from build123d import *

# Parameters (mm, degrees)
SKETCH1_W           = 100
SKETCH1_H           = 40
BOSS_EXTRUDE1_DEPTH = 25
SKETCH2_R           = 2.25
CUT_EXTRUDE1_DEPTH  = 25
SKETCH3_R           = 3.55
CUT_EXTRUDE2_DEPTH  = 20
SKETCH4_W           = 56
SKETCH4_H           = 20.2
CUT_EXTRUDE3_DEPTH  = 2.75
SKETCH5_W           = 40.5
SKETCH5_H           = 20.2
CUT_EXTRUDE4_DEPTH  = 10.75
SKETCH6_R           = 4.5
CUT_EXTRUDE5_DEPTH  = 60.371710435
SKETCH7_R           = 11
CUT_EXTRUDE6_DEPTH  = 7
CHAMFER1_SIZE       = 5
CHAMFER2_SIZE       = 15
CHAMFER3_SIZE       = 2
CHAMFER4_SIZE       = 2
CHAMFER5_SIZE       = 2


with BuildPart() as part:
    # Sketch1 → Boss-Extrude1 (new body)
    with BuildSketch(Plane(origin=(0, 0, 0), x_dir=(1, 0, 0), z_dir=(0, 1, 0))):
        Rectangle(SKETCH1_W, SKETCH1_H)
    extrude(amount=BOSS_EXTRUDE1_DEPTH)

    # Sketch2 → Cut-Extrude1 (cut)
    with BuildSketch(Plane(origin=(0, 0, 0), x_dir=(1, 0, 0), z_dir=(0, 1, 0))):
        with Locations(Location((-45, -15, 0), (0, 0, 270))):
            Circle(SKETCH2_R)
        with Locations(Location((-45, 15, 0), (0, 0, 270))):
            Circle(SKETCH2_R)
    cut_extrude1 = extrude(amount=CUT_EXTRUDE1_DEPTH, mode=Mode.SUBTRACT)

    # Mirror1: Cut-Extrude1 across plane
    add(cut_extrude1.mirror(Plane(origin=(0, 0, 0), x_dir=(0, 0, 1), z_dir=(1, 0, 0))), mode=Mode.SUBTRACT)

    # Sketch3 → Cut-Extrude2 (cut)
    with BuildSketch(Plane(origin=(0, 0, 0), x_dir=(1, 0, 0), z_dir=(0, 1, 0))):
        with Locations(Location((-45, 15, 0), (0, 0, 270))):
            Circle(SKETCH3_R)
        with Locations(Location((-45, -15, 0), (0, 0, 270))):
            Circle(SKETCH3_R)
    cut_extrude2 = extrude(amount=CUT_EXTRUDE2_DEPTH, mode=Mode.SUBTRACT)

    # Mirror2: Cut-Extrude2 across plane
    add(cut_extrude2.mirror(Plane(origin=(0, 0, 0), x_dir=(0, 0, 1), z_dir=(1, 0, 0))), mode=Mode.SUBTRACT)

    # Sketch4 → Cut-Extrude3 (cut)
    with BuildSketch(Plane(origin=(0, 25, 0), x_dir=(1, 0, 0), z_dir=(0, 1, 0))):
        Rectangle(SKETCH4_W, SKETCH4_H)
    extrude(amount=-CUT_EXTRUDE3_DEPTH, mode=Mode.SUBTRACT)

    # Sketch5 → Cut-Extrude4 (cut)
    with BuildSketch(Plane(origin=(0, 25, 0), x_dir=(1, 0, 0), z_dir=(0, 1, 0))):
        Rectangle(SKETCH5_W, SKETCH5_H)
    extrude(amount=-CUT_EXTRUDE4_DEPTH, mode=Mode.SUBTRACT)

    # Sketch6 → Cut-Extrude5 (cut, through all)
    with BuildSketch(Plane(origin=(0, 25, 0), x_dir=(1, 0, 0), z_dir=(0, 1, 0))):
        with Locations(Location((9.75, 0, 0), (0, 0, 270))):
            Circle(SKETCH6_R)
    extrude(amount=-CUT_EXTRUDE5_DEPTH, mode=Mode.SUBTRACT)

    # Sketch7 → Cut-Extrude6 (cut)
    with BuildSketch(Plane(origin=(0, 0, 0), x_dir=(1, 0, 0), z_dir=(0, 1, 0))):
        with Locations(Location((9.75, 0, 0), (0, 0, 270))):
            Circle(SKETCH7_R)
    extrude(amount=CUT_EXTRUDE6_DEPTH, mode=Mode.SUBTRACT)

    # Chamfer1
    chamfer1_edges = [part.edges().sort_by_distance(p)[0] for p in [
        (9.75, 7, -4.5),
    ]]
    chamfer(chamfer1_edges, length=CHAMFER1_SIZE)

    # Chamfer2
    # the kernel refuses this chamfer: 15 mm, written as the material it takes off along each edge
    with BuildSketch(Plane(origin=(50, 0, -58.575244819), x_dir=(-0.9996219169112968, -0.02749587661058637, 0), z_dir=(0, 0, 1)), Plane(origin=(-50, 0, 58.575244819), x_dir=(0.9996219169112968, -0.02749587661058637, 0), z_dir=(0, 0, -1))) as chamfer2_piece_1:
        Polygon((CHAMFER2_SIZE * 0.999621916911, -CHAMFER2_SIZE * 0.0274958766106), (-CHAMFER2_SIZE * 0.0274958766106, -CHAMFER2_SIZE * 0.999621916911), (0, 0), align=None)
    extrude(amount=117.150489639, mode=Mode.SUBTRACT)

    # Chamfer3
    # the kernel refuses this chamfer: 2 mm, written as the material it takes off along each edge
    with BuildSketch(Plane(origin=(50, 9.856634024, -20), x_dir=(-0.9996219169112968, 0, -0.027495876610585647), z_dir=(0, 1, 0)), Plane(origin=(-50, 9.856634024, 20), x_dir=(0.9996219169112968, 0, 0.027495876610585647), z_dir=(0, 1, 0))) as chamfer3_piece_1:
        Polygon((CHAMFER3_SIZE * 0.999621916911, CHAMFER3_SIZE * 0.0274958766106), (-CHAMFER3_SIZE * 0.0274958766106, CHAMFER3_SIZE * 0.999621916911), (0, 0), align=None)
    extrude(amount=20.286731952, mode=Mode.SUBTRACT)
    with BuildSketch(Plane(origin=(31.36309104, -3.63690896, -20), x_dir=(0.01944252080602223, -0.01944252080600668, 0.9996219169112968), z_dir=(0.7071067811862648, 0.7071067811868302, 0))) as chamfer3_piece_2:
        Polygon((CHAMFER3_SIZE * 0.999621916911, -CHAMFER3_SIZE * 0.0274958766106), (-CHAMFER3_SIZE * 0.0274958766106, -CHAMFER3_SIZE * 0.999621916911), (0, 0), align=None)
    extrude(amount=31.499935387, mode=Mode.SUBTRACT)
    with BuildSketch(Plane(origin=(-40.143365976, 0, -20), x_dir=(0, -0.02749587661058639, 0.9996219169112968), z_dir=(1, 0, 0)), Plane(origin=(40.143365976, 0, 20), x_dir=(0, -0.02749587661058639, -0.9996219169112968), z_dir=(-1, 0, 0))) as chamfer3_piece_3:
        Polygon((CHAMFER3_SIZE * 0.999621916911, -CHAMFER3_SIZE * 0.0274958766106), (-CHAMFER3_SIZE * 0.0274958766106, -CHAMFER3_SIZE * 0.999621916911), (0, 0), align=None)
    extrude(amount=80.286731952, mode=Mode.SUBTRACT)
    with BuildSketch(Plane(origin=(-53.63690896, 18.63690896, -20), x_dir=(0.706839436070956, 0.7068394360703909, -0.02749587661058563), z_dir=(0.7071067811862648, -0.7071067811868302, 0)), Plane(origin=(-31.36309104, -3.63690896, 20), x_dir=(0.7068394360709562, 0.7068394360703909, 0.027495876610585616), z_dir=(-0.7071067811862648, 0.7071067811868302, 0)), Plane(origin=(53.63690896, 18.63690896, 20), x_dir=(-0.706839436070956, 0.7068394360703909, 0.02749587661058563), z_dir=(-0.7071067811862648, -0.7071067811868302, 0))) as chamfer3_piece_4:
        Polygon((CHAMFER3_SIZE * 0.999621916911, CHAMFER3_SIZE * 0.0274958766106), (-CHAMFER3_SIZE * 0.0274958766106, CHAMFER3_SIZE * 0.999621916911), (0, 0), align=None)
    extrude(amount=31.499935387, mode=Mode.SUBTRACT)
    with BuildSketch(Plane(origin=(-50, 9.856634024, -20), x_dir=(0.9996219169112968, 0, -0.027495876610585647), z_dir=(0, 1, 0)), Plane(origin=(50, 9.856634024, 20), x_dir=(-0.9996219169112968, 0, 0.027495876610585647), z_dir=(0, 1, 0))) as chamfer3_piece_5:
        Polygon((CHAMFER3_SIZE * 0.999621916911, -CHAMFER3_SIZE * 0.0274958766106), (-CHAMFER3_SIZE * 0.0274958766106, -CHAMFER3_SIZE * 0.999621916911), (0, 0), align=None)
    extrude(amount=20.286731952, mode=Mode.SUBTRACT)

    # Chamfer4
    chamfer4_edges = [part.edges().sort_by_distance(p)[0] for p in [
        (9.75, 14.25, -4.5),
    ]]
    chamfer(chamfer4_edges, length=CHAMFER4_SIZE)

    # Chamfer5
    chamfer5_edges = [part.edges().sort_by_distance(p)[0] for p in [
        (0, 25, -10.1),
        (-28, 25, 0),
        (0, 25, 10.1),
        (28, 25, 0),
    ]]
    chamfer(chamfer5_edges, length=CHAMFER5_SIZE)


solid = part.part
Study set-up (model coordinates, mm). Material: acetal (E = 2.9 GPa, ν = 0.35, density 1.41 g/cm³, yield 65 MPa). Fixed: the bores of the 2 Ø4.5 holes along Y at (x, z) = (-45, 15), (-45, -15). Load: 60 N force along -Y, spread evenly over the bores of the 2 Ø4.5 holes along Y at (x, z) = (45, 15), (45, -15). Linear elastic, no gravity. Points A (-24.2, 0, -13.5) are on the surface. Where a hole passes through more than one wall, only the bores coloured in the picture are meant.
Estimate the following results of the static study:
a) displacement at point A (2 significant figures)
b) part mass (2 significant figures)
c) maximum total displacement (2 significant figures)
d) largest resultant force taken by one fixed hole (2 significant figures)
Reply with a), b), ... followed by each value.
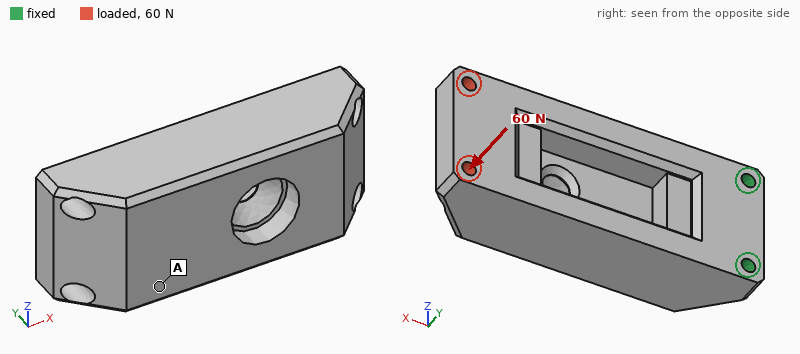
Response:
a) 0.37 mm
b) 110 g
c) 1.3 mm
d) 33 N
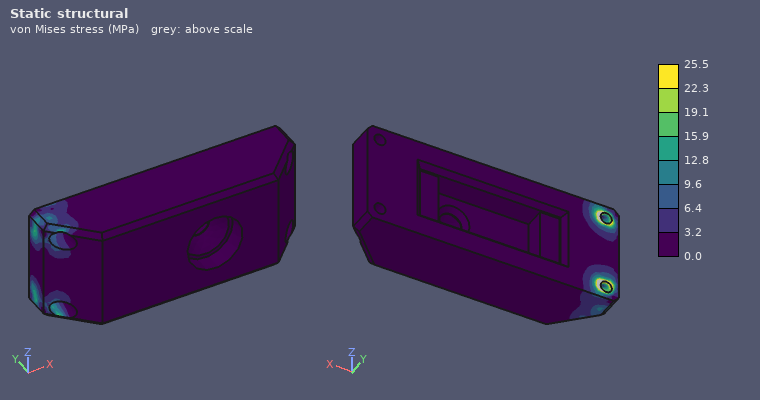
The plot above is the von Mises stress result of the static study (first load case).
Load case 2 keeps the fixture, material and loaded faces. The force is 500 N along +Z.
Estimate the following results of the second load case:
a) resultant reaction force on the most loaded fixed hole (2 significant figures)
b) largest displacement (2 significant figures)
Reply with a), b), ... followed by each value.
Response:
a) 1.4 kN
b) 1.2 mm
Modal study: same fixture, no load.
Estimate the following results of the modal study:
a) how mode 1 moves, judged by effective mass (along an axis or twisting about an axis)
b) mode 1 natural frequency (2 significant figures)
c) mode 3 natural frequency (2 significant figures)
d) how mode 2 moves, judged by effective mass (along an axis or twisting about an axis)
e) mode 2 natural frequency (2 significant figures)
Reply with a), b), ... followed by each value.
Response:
a) along Y
b) 190 Hz
c) 1400 Hz
d) along Z
e) 640 Hz
